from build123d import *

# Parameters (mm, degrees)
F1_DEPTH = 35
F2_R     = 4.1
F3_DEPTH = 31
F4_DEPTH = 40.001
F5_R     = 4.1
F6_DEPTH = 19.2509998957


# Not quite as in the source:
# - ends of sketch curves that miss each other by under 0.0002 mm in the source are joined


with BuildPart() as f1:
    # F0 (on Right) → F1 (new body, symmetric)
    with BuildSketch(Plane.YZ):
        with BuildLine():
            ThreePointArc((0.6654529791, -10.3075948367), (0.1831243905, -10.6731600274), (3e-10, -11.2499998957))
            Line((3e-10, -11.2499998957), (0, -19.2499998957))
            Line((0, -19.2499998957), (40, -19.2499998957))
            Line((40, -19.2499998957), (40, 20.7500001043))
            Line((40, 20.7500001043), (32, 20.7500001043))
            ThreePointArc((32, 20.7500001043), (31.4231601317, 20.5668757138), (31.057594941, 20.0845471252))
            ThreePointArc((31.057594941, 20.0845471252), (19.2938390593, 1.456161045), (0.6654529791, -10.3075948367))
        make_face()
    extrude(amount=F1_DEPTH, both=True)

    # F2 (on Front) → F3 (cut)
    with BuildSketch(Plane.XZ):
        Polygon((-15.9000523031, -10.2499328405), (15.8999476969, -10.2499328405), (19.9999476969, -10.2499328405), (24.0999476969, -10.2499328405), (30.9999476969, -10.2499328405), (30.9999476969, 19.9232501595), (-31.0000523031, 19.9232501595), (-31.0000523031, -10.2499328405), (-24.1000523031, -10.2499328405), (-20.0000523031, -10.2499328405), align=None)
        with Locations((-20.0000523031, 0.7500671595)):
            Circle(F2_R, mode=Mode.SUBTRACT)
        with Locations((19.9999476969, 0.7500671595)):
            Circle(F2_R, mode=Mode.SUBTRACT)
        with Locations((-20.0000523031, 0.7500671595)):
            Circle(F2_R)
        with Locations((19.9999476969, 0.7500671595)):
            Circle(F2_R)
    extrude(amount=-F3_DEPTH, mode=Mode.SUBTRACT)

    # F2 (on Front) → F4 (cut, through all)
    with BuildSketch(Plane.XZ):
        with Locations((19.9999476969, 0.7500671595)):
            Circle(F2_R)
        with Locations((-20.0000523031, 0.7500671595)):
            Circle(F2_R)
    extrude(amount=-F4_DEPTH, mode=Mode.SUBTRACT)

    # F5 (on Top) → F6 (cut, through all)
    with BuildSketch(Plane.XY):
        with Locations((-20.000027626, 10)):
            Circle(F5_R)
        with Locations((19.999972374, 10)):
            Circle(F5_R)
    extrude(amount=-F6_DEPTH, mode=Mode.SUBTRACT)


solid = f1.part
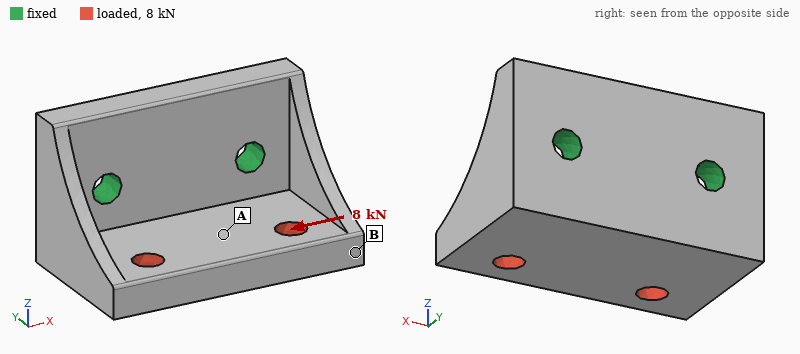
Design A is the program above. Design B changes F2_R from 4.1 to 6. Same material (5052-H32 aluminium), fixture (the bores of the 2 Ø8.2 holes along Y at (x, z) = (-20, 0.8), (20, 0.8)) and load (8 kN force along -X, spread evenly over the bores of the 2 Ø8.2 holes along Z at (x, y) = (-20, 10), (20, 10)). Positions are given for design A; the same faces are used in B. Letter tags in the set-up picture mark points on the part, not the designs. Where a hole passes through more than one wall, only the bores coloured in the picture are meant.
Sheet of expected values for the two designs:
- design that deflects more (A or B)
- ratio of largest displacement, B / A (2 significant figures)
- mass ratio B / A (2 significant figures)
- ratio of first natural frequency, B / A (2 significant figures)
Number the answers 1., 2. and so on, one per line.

1. A
2. 0.76
3. 0.98
4. 1.1
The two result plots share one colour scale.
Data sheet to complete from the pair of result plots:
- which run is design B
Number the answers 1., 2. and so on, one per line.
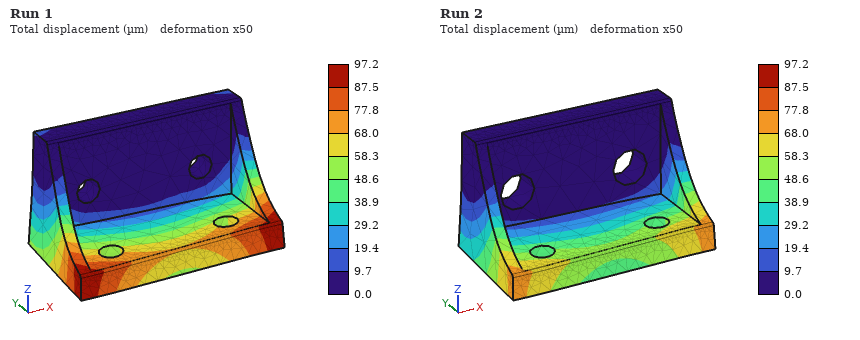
1. Run 2
